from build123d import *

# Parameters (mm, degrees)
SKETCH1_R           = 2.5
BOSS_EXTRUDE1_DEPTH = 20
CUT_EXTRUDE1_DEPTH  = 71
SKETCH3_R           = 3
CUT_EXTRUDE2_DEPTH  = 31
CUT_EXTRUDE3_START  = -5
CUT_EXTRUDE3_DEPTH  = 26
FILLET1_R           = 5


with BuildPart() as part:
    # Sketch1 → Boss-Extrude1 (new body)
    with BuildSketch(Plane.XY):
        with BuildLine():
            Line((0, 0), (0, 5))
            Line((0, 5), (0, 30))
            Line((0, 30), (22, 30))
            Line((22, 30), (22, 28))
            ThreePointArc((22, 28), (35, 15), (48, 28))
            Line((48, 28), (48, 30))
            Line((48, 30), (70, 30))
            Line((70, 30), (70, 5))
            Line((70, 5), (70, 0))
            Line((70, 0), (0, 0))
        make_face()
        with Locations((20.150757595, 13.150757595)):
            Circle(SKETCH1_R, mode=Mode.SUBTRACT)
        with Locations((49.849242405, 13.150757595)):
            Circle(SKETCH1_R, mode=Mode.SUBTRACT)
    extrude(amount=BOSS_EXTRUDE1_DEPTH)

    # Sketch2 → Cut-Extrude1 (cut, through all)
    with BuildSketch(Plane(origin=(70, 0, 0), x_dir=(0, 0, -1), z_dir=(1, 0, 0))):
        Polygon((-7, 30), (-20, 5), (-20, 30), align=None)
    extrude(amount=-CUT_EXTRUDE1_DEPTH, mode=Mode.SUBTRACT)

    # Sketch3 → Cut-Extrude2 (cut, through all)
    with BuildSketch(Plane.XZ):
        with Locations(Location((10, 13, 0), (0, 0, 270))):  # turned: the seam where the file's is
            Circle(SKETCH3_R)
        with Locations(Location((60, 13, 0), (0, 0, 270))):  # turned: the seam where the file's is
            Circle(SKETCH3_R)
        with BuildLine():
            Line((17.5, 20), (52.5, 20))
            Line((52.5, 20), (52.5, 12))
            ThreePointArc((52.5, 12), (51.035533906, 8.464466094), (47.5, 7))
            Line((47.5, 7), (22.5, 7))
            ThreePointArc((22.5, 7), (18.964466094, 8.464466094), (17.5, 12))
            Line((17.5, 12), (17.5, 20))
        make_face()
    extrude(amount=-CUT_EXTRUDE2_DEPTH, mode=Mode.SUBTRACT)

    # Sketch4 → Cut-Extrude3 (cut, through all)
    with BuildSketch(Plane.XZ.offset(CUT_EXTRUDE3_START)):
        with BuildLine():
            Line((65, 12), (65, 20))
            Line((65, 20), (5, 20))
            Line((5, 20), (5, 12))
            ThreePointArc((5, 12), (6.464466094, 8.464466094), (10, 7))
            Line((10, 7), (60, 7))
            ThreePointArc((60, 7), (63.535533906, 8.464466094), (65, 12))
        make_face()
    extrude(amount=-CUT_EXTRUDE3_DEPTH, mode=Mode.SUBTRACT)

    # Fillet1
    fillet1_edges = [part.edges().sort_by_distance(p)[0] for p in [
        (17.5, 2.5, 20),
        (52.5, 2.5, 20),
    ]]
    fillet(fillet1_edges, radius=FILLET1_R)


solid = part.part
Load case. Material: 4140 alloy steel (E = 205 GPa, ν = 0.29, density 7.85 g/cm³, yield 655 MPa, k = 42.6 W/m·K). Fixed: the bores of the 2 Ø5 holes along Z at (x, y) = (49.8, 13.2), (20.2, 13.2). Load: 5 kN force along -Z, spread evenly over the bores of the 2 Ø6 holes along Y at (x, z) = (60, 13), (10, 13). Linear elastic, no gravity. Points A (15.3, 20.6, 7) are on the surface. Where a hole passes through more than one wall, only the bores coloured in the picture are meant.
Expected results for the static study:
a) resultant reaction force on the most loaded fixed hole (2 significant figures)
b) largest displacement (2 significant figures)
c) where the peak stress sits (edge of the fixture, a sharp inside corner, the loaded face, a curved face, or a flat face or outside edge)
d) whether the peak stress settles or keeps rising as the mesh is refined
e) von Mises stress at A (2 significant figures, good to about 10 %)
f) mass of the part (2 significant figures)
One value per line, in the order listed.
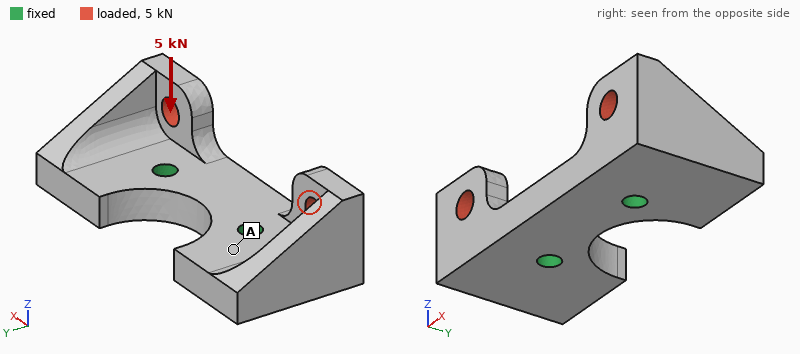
2.5 kN
48 µm
edge of the fixture
keeps rising
50 MPa
130 g
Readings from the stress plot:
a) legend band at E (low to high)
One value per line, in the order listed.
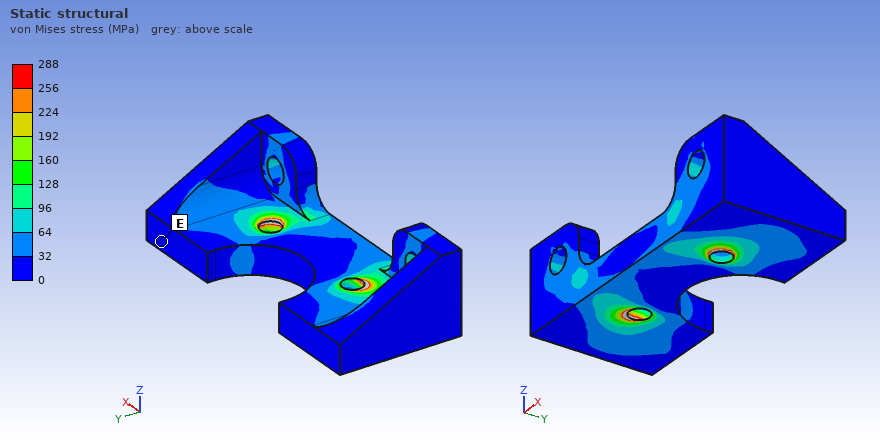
0 to 32 MPa
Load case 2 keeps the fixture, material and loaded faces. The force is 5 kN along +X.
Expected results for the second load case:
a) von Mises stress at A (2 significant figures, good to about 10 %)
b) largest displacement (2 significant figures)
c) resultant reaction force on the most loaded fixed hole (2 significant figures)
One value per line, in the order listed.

37 MPa
45 µm
2.8 kN
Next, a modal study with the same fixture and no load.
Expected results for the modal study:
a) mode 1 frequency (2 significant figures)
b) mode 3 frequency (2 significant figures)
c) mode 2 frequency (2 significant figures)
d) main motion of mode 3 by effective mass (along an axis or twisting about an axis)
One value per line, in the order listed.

7900 Hz
9700 Hz
8000 Hz
along Y
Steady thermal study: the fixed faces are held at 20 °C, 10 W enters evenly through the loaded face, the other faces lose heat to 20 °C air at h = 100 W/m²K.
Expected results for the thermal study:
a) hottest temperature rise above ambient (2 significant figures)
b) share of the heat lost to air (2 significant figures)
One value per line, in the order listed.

17 K
32 %
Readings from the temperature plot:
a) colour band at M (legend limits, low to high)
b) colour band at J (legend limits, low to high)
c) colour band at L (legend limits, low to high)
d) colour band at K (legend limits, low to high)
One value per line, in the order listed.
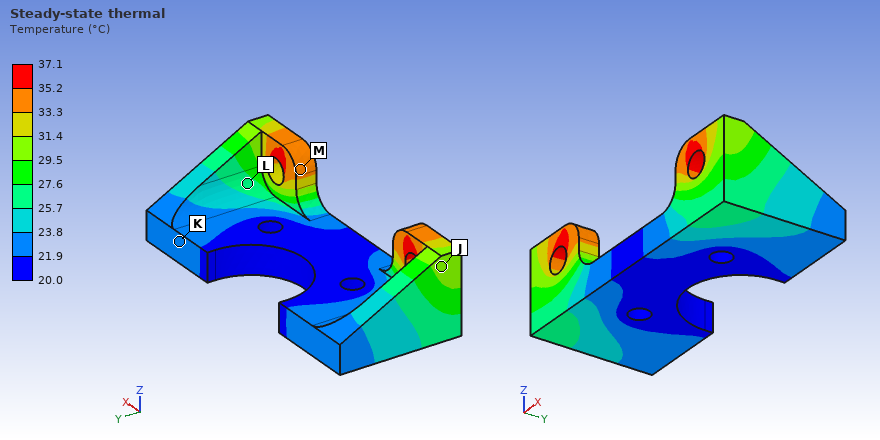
33.3 to 35.2 °C
29.5 to 31.4 °C
25.7 to 27.6 °C
21.9 to 23.8 °C
